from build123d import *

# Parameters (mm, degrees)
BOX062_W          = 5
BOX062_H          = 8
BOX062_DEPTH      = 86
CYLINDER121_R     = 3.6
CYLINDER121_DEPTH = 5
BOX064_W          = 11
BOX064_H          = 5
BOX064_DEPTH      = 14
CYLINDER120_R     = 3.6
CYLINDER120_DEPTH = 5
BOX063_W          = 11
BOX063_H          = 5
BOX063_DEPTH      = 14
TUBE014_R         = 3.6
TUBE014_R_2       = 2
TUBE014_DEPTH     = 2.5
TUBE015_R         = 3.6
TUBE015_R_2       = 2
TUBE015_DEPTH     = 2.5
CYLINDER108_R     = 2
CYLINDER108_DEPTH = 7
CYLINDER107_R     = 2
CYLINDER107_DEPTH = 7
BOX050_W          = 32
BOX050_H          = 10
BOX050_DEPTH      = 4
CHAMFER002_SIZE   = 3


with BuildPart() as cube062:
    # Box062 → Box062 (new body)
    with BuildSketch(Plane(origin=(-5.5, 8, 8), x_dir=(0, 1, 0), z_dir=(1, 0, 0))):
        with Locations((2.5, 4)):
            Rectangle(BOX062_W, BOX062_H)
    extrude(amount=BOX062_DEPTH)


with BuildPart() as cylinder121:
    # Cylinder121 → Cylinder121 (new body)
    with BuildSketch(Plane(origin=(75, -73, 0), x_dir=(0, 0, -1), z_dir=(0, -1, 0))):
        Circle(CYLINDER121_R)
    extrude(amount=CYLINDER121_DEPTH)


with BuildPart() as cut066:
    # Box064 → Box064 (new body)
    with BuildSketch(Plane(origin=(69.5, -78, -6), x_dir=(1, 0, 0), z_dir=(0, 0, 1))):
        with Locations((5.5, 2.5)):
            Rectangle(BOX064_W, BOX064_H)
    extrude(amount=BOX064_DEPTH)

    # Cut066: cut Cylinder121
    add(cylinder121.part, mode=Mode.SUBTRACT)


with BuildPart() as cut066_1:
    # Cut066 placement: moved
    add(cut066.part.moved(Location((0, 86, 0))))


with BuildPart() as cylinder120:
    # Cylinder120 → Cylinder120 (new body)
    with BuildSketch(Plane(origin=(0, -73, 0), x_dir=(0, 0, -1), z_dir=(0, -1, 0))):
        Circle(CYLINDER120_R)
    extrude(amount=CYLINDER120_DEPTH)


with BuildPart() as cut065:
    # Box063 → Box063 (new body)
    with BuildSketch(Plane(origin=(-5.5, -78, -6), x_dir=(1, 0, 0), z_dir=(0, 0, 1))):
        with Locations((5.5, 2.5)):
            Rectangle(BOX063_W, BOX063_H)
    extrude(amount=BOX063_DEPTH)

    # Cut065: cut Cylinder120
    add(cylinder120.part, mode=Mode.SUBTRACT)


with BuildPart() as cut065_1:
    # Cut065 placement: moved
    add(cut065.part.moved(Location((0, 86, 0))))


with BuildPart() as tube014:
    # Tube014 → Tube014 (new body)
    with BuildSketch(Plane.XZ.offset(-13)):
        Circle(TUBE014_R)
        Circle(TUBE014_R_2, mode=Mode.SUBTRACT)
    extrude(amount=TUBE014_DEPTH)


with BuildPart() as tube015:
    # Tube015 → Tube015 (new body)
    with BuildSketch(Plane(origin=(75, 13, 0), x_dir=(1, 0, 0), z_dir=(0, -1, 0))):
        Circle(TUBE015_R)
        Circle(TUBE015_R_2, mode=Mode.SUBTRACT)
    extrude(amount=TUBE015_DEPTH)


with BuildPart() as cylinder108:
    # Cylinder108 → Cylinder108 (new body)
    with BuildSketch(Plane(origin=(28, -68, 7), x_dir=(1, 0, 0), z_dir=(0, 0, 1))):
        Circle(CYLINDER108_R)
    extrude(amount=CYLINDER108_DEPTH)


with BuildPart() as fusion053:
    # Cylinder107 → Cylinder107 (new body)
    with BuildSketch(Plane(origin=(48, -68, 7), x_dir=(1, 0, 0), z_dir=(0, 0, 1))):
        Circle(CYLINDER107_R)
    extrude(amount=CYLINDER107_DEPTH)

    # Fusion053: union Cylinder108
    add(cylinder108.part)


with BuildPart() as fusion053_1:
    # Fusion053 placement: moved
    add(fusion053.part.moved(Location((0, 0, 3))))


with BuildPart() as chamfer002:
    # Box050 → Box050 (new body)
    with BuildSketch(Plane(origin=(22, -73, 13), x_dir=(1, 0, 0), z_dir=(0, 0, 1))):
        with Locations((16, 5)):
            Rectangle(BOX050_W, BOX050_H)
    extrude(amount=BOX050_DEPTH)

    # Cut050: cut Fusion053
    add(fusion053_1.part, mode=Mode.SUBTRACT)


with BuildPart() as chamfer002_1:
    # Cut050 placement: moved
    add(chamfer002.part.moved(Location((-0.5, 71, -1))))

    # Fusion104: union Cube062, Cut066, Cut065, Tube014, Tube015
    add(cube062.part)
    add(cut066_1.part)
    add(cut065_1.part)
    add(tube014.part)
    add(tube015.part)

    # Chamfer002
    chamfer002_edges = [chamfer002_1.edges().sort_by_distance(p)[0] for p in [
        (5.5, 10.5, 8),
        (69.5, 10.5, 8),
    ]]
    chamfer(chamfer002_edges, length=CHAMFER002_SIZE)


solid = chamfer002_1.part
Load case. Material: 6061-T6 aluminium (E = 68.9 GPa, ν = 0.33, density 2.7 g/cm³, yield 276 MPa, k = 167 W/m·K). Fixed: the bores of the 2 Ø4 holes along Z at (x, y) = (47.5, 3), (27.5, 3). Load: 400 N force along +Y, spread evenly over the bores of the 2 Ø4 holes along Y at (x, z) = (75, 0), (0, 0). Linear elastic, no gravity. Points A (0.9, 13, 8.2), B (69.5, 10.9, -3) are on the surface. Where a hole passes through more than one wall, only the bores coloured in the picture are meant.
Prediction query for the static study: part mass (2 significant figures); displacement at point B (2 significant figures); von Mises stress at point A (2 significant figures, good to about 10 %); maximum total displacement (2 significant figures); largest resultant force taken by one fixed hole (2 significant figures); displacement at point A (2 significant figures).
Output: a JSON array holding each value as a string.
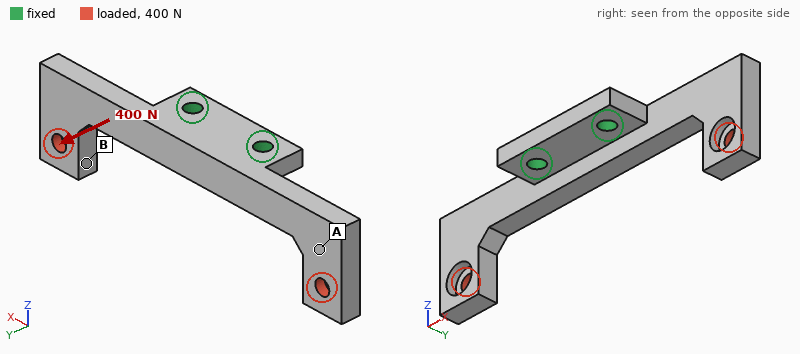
["16 g", "0.35 mm", "30 MPa", "0.53 mm", "500 N", "0.26 mm"]
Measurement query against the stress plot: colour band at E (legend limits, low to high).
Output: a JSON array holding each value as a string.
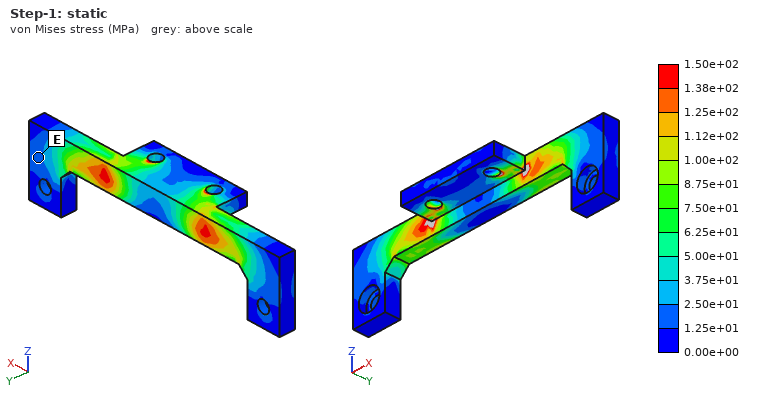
["1.25e+01 to 2.50e+01 MPa"]
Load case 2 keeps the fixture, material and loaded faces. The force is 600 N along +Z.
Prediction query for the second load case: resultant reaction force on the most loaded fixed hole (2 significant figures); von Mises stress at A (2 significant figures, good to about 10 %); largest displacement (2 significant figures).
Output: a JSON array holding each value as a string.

["420 N", "16 MPa", "0.34 mm"]
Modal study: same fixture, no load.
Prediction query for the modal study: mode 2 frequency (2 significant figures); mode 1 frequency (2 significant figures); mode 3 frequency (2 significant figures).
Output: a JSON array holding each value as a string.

["2400 Hz", "2400 Hz", "3100 Hz"]
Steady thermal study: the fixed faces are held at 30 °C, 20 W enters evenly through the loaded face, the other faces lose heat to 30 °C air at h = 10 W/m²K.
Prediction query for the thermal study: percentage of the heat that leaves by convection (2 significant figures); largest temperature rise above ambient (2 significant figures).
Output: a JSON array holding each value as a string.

["4.8 %", "53 K"]
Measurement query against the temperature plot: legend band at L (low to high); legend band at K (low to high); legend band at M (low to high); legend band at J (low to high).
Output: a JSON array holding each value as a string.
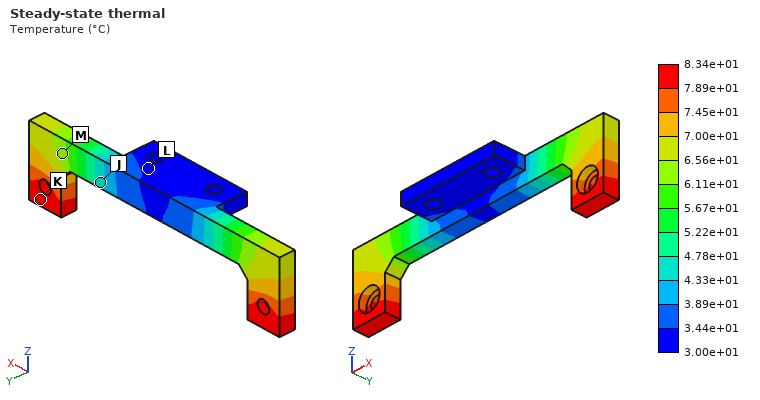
["3.00e+01 to 3.44e+01 °C", "7.89e+01 to 8.34e+01 °C", "6.11e+01 to 6.56e+01 °C", "4.33e+01 to 4.78e+01 °C"]
